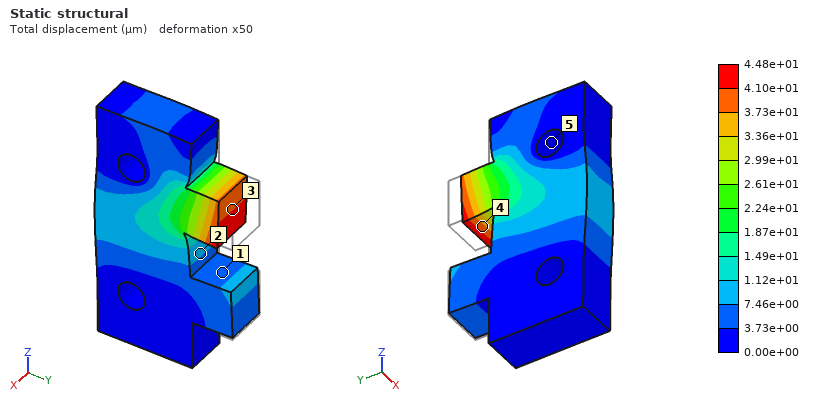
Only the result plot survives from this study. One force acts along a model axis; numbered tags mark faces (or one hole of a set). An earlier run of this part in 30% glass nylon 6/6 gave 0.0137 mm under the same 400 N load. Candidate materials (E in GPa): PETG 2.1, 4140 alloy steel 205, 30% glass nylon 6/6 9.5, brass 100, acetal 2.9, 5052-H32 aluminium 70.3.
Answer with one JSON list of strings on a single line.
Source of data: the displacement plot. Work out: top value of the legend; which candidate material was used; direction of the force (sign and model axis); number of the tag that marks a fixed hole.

["4.48e+01 µm", "acetal", "-Y", "5"]
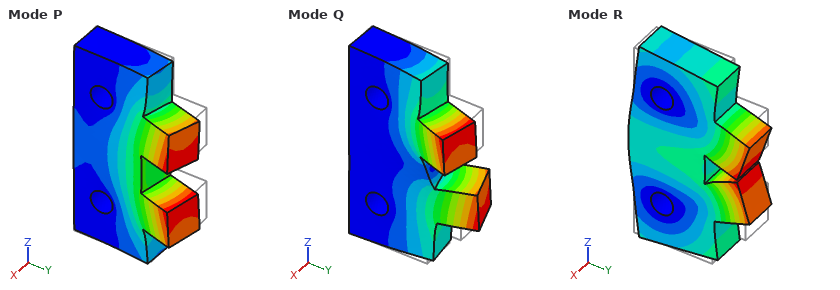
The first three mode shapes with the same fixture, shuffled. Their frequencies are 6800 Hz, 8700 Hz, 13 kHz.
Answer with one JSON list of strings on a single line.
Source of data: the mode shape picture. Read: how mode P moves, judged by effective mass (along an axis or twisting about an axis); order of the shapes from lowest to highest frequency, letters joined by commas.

["along X", "P, Q, R"]
